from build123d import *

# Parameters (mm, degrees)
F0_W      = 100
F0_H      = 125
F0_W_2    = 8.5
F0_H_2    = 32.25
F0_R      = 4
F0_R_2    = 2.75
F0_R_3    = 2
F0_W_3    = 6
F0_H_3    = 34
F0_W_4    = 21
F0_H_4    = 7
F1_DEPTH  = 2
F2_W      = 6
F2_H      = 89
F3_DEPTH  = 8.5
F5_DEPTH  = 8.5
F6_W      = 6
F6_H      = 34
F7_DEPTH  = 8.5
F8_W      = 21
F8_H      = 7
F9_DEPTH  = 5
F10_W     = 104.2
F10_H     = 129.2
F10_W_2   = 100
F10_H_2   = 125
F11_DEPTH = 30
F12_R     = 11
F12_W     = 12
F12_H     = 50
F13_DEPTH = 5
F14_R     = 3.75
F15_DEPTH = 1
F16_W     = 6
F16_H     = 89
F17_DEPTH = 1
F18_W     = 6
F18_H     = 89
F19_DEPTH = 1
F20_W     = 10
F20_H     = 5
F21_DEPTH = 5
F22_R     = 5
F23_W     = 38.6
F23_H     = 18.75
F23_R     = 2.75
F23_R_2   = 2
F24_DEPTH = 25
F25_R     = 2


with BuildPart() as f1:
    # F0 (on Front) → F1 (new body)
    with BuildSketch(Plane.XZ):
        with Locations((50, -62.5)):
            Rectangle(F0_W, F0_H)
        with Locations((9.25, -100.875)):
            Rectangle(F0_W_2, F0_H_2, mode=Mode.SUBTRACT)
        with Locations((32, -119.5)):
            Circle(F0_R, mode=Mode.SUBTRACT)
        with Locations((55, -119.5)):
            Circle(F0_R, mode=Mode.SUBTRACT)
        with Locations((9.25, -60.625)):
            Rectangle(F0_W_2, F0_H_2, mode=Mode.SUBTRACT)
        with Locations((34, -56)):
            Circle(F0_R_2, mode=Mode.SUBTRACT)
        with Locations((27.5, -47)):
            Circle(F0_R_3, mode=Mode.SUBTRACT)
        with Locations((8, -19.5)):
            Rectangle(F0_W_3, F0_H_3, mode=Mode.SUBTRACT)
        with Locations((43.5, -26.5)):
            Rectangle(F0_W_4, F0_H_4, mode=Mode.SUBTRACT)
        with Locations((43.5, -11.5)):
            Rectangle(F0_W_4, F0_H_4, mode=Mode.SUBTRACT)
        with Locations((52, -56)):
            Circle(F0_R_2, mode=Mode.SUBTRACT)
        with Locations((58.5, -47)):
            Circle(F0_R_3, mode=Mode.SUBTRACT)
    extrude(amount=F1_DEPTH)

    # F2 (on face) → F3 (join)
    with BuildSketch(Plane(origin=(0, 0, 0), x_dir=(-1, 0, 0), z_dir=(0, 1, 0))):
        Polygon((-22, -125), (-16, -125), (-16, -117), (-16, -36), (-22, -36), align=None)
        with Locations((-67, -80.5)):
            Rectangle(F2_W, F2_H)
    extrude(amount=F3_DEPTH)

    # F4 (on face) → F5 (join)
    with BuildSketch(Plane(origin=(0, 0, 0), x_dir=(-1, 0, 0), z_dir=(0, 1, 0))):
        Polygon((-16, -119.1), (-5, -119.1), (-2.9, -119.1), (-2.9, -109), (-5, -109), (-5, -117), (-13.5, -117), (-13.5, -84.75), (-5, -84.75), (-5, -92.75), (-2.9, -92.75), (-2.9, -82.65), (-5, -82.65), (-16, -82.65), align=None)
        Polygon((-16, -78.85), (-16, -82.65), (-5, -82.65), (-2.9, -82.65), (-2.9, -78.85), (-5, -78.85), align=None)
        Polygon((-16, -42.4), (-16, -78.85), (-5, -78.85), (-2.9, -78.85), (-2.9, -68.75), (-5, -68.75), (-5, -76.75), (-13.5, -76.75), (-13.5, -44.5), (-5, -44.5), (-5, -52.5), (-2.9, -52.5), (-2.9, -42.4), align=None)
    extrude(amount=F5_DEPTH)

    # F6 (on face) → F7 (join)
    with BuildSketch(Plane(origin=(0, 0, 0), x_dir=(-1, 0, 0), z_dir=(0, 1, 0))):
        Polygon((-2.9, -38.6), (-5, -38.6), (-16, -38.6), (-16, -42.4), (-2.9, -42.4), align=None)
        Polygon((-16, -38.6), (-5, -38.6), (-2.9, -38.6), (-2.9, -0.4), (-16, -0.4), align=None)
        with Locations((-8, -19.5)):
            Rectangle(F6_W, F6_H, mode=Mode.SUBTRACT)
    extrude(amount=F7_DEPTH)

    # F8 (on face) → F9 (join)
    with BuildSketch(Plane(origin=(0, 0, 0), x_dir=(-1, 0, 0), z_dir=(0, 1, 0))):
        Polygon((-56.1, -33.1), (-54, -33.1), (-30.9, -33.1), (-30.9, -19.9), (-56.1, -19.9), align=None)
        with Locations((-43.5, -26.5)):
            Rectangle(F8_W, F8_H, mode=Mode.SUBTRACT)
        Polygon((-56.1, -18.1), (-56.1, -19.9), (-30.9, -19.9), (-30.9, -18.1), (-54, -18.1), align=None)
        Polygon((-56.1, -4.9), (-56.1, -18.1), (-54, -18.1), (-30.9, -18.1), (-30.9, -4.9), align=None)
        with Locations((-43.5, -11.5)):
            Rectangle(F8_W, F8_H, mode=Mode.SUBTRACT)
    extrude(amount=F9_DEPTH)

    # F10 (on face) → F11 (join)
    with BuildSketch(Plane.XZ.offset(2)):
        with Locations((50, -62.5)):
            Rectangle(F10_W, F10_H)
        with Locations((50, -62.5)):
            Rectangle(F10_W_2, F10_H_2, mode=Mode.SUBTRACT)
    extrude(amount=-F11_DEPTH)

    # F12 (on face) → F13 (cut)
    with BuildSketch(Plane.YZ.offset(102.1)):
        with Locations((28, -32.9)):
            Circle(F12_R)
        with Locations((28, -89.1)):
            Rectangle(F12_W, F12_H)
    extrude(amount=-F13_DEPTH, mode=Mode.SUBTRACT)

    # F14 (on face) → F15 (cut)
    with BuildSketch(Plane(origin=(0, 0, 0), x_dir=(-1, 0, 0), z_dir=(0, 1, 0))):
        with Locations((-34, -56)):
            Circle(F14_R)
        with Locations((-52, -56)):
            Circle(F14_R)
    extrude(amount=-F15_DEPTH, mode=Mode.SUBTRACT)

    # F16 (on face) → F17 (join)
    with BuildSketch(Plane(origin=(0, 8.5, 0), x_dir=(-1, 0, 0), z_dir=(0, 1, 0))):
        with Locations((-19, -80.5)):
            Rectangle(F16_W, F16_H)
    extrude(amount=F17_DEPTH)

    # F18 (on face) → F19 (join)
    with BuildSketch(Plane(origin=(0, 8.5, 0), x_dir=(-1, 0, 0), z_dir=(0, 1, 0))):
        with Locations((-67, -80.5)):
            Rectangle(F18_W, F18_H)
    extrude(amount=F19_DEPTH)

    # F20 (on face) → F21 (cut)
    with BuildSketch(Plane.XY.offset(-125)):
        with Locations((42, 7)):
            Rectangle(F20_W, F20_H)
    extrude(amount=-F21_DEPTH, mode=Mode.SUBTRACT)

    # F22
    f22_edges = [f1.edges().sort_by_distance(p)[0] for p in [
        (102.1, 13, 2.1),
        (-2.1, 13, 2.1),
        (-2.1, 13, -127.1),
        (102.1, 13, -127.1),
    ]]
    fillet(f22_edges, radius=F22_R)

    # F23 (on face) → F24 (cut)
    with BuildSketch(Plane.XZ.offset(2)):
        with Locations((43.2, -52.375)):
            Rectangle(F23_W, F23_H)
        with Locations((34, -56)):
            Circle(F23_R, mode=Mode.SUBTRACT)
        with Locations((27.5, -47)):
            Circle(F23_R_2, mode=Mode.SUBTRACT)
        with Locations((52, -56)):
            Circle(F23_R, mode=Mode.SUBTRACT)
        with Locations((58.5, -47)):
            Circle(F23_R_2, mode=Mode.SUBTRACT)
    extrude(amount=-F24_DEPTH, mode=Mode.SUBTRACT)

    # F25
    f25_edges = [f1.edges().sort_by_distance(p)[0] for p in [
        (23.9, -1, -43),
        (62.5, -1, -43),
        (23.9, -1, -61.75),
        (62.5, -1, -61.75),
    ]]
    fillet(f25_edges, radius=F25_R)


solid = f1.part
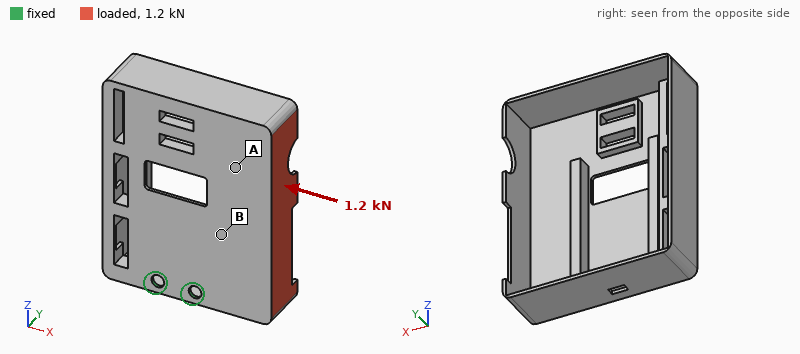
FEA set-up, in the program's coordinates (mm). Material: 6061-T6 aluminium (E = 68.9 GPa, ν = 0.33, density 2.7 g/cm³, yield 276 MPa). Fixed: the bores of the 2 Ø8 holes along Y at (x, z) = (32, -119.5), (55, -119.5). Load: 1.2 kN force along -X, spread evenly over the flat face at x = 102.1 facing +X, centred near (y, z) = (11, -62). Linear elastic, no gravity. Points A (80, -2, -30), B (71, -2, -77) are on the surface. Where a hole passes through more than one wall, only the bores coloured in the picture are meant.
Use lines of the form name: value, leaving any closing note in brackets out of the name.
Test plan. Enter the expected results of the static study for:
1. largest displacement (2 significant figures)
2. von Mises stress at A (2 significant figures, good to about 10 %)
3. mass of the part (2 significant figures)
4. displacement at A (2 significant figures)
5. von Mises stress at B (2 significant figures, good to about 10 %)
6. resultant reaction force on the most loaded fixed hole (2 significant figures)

largest displacement: 1.7 mm
von Mises stress at A: 43 MPa
mass of the part: 180 g
displacement at A: 0.51 mm
von Mises stress at B: 17 MPa
resultant reaction force on the most loaded fixed hole: 2.3 kN
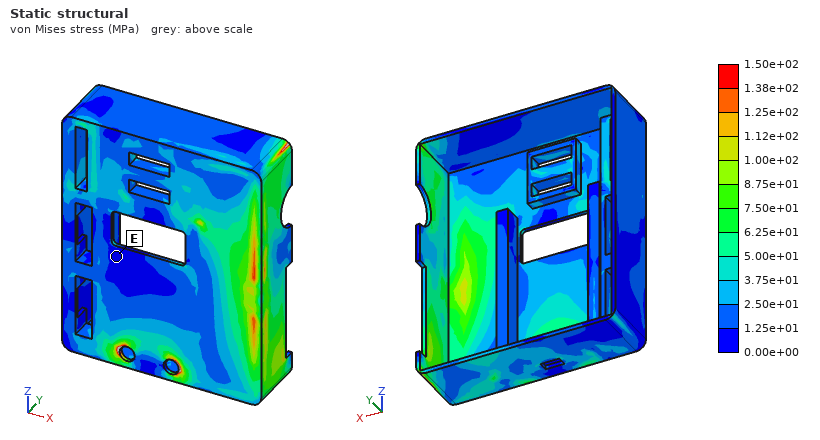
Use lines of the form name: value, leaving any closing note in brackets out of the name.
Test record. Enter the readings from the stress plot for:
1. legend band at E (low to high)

legend band at E: 0.00e+00 to 1.25e+01 MPa
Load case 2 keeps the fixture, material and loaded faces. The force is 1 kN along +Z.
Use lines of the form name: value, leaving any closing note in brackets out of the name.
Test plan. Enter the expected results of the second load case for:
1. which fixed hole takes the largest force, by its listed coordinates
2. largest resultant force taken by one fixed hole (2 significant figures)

which fixed hole takes the largest force, by its listed coordinates: (55, -119.5)
largest resultant force taken by one fixed hole: 2.4 kN
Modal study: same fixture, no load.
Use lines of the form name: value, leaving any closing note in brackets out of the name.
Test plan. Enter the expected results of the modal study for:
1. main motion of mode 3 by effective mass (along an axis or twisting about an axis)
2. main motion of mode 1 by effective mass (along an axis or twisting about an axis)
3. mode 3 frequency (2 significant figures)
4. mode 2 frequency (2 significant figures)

main motion of mode 3 by effective mass: along X
main motion of mode 1 by effective mass: along Y
mode 3 frequency: 1100 Hz
mode 2 frequency: 360 Hz
